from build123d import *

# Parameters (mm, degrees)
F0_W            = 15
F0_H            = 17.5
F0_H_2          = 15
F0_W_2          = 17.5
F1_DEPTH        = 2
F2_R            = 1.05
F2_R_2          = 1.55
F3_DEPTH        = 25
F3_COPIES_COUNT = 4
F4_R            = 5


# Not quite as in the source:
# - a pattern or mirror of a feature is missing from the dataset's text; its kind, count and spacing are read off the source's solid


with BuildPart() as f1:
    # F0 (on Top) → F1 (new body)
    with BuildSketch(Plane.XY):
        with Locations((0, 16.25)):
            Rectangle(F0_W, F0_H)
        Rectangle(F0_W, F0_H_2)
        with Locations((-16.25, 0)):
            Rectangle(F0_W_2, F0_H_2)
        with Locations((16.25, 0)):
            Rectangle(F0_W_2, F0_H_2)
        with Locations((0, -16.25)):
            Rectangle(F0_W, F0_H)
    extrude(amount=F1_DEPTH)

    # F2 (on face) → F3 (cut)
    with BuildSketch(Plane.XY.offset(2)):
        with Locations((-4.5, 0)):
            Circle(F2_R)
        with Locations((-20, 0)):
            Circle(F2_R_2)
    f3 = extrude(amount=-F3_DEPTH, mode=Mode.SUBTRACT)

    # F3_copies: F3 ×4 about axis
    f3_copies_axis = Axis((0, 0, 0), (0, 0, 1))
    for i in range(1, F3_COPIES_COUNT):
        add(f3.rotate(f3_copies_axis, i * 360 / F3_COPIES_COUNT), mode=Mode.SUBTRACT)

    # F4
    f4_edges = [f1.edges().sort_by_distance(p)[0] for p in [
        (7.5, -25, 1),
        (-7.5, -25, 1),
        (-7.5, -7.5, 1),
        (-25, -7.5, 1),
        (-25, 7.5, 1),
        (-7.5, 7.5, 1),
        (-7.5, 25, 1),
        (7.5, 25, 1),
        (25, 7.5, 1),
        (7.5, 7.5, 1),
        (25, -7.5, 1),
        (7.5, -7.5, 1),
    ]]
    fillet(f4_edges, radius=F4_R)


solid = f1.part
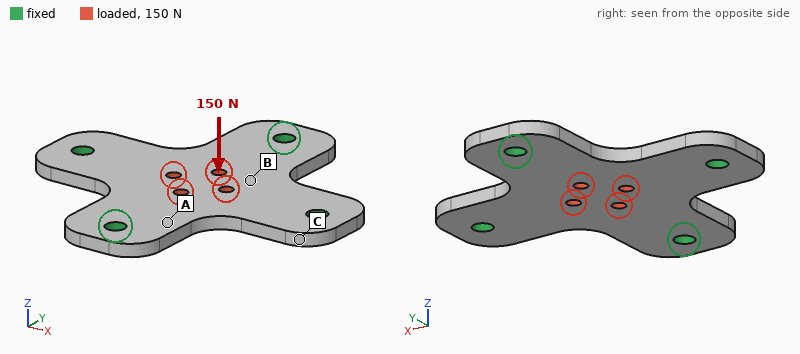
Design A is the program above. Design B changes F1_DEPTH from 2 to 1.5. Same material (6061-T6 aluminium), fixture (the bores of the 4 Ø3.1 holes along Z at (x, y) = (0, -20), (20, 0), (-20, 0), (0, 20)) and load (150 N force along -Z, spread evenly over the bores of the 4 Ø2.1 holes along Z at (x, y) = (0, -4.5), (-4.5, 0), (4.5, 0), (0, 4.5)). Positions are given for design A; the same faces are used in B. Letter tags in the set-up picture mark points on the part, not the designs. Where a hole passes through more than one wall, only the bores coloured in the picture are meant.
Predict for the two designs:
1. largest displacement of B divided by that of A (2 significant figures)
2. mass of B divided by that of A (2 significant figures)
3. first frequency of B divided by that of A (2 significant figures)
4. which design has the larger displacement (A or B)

2.3
0.75
0.77
B
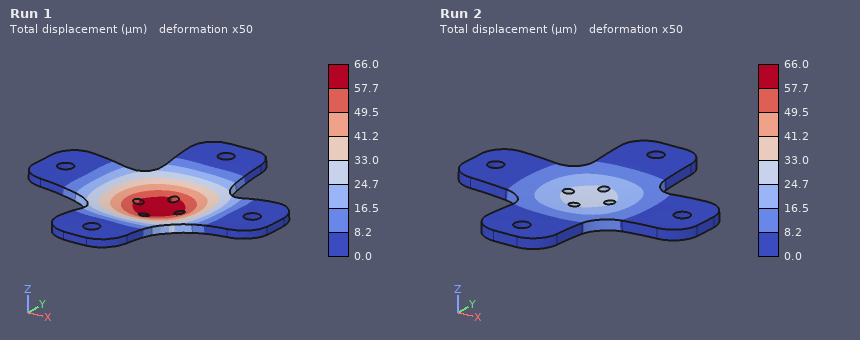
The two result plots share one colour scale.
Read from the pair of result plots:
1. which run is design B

Run 1
